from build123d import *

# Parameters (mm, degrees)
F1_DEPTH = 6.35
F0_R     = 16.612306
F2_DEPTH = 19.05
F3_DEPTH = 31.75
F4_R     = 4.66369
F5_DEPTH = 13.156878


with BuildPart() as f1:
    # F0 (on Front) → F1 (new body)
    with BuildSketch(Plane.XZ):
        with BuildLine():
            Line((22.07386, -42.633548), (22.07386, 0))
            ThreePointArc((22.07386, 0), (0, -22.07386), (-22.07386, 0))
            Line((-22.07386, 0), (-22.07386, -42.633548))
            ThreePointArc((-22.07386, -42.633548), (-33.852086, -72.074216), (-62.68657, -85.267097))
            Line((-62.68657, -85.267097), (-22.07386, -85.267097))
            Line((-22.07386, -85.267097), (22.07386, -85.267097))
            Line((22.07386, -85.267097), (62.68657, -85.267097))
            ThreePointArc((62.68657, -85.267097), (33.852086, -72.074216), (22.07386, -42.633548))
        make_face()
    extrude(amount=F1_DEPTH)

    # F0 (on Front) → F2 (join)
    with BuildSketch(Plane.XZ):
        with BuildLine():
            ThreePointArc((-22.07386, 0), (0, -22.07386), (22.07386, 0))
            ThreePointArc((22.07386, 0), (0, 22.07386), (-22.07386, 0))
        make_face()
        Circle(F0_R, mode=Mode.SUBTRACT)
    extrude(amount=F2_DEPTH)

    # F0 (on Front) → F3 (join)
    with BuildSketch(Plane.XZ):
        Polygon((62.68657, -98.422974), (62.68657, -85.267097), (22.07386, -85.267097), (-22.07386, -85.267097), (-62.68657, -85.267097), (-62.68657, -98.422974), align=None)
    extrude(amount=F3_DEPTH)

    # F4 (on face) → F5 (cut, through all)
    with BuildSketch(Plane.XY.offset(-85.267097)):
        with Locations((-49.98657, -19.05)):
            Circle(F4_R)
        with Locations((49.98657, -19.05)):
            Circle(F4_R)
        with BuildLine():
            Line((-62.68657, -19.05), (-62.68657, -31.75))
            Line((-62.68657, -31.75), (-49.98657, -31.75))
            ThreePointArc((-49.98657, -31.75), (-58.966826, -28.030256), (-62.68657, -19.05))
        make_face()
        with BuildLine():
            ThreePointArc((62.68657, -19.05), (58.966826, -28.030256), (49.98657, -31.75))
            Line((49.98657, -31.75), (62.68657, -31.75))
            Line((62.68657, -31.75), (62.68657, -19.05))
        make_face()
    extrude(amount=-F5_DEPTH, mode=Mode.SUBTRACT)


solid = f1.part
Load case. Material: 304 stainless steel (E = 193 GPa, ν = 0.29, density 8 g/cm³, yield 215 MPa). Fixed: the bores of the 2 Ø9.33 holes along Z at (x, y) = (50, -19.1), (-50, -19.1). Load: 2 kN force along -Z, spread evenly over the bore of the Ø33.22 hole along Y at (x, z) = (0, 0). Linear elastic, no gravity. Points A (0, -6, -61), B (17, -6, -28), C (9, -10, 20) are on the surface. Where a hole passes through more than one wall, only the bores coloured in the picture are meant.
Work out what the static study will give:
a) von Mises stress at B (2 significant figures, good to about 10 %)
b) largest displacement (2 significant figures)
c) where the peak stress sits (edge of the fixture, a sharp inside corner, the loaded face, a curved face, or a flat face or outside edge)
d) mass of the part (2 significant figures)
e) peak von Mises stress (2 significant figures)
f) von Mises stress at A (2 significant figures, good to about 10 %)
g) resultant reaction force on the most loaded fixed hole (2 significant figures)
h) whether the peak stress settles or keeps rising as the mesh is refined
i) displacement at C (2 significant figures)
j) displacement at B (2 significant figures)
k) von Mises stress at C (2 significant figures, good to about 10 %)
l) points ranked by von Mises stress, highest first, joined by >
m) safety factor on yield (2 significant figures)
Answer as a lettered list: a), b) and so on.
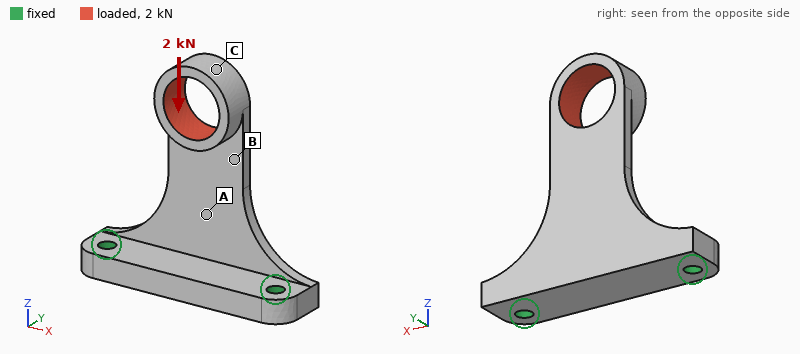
a) 50 MPa
b) 0.31 mm
c) a curved face
d) 690 g
e) 57 MPa
f) 37 MPa
g) 1.1 kN
h) settles
i) 0.30 mm
j) 0.091 mm
k) 9.8 MPa
l) B > A > C
m) 3.7
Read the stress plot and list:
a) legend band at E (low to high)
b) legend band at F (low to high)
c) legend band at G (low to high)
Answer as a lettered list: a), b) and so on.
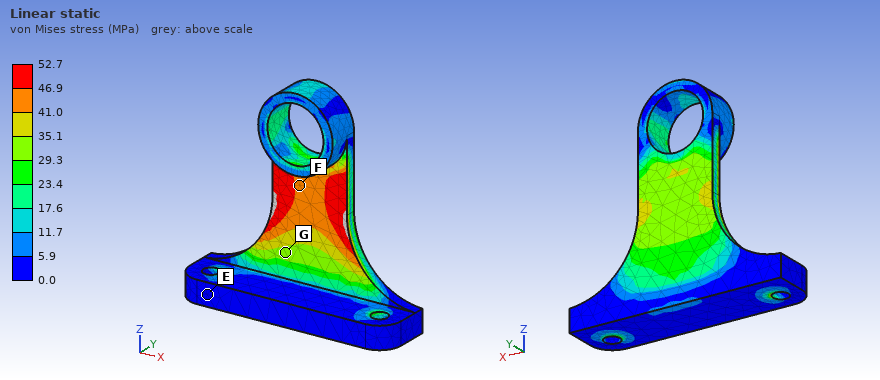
a) 0.0 to 5.9 MPa
b) 41.0 to 46.9 MPa
c) 29.3 to 35.1 MPa
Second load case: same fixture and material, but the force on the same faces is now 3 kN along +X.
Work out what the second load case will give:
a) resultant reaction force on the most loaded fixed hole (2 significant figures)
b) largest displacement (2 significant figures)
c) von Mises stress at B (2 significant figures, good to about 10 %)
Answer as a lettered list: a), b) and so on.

a) 3.5 kN
b) 0.19 mm
c) 65 MPa
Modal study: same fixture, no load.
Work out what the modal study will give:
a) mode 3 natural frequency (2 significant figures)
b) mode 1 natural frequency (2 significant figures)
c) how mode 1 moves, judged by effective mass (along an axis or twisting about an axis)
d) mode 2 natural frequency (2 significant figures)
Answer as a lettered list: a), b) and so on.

a) 2400 Hz
b) 440 Hz
c) along Y
d) 1800 Hz
